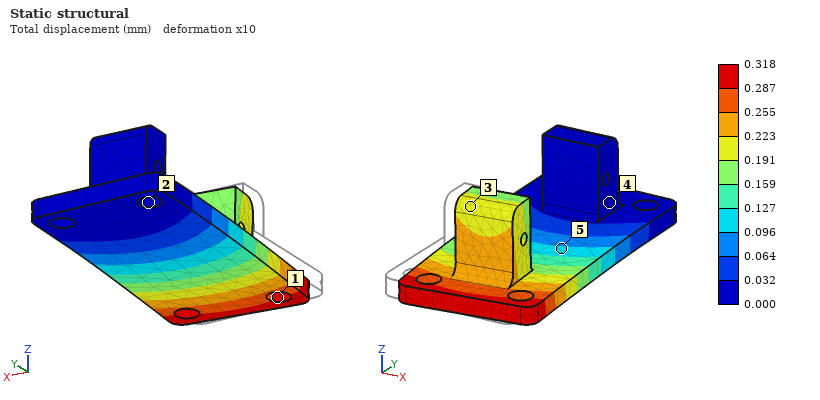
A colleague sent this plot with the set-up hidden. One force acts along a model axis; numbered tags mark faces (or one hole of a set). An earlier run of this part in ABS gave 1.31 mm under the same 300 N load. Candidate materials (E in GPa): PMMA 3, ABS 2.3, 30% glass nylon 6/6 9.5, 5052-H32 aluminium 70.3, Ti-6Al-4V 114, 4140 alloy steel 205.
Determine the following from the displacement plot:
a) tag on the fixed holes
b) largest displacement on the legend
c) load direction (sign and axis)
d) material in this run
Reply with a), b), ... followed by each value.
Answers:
a) 2
b) 0.318 mm
c) +X
d) 30% glass nylon 6/6
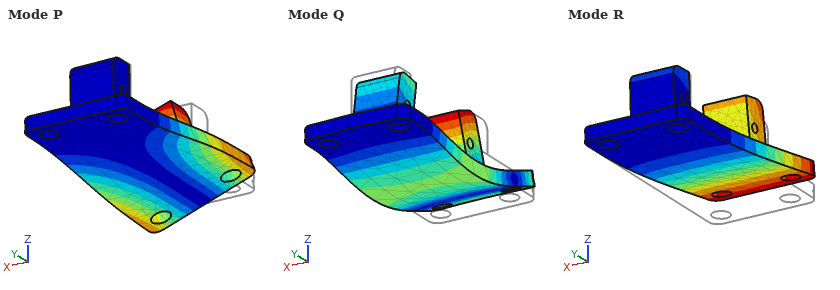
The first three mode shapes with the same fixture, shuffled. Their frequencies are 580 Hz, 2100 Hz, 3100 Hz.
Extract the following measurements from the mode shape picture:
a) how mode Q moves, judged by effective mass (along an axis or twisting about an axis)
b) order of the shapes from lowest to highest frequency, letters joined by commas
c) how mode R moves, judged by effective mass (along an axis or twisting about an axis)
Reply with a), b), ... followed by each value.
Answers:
a) along Z
b) R, P, Q
c) along Z
